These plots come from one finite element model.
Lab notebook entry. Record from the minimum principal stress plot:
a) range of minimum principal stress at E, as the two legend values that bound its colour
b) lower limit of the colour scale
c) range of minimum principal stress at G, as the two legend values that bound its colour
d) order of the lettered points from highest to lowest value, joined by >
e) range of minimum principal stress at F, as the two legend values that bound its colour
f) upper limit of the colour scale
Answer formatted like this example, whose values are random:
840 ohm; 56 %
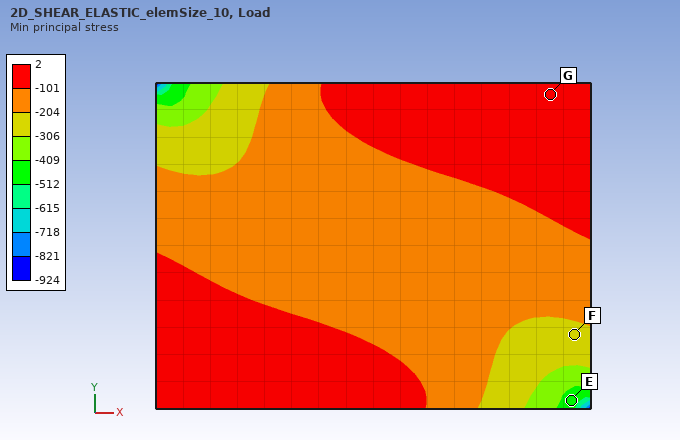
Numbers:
-512 to -409; -924; -101 to 2; G > F > E; -306 to -204; 2
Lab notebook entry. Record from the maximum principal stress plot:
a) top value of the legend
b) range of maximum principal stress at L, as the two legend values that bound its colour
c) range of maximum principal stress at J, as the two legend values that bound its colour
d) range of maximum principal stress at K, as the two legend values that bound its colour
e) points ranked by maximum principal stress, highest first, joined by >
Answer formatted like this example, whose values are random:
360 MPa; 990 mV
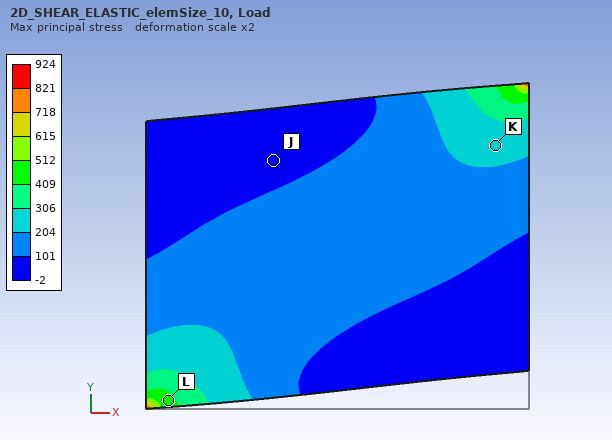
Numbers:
924; 409 to 512; -2 to 101; 204 to 306; L > K > J
